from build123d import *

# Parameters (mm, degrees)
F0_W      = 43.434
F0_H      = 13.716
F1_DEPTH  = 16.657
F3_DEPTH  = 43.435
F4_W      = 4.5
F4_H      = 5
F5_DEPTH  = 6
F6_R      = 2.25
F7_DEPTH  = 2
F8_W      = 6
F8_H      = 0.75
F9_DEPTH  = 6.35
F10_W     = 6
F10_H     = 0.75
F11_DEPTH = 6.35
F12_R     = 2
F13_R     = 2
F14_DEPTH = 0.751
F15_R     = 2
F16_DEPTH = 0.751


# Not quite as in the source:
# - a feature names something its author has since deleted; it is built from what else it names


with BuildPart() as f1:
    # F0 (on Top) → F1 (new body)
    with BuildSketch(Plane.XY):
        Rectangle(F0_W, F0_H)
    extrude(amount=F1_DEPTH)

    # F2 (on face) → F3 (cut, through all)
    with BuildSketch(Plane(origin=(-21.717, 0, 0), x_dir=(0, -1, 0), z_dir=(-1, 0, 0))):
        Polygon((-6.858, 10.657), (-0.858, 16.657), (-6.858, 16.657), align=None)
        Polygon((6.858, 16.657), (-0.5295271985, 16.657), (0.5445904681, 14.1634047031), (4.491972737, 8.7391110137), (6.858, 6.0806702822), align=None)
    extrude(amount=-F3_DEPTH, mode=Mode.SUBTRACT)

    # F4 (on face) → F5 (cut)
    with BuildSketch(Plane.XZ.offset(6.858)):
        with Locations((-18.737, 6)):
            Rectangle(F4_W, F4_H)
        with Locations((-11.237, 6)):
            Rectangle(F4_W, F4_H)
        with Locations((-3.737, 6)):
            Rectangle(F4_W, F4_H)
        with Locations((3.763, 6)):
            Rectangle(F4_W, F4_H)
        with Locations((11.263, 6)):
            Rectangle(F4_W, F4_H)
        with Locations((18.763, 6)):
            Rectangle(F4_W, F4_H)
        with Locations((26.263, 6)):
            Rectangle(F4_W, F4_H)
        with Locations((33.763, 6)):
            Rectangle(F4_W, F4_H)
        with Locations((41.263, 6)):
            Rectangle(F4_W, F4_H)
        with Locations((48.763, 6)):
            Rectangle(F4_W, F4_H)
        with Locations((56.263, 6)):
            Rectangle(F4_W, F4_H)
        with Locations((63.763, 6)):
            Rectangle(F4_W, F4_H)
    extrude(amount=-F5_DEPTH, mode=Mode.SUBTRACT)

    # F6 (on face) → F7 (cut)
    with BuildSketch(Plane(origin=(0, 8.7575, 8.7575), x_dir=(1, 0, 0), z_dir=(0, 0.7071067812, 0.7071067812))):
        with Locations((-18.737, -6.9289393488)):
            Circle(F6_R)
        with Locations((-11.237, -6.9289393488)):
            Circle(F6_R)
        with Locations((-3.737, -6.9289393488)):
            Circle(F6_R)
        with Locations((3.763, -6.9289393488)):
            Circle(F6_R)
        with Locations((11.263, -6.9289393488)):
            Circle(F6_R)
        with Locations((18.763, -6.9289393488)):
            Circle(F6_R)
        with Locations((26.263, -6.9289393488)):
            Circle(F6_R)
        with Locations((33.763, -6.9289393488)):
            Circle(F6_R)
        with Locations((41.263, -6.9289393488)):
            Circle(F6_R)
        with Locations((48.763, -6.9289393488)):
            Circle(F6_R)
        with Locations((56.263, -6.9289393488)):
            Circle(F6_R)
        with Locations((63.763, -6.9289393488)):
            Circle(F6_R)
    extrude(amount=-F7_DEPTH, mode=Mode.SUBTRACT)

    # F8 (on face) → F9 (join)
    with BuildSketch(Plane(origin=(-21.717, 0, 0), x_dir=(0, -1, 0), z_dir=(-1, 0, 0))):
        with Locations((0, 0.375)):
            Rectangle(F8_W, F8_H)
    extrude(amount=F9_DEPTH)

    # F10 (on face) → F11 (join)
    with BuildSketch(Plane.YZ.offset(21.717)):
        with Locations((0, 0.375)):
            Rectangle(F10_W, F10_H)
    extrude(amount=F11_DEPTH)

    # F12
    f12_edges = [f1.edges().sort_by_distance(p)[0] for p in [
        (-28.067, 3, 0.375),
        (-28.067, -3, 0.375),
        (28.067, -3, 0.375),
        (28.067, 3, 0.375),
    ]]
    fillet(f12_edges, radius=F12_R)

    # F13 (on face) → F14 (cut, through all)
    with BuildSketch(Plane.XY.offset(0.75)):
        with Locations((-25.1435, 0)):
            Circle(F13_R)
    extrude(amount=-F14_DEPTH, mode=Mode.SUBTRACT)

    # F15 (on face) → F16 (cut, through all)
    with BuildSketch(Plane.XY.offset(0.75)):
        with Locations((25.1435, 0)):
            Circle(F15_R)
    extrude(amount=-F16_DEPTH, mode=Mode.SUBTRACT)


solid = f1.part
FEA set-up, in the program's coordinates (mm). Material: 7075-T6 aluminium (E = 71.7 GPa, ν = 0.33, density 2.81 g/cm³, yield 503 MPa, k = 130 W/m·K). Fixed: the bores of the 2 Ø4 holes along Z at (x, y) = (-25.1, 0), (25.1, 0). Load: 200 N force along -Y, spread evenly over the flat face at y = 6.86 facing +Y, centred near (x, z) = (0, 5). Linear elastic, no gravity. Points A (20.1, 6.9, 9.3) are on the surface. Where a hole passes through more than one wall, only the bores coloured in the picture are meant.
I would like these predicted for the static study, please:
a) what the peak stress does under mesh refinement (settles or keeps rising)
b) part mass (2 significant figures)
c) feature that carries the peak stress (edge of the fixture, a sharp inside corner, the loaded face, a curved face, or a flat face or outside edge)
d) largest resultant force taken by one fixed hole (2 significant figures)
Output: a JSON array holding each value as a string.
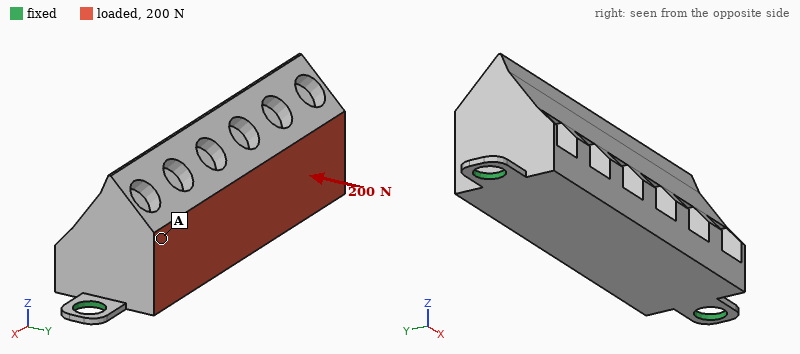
["keeps rising", "18 g", "edge of the fixture", "100 N"]
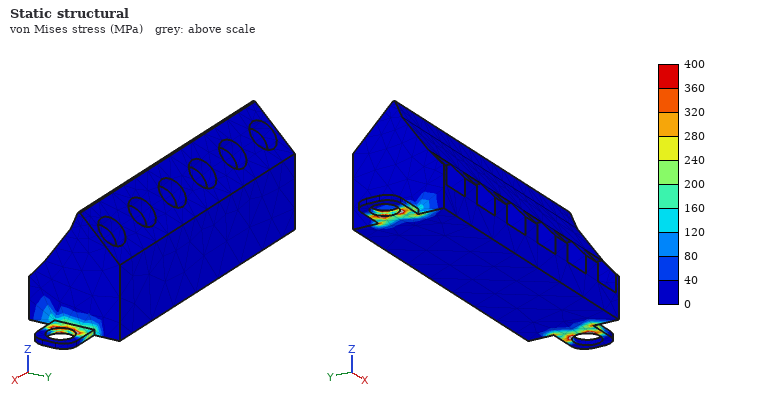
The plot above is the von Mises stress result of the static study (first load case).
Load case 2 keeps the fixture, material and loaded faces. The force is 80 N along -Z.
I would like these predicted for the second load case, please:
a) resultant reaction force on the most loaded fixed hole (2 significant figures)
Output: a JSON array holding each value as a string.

["50 N"]
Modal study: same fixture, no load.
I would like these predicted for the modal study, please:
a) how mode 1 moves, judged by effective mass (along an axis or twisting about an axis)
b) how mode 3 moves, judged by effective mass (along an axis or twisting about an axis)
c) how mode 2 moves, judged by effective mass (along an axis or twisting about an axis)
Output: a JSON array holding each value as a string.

["along Y", "along X", "along Z"]
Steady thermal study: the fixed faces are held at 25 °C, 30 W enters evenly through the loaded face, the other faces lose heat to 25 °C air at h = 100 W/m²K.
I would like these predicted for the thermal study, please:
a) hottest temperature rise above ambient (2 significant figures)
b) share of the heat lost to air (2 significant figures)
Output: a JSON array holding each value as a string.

["50 K", "43 %"]
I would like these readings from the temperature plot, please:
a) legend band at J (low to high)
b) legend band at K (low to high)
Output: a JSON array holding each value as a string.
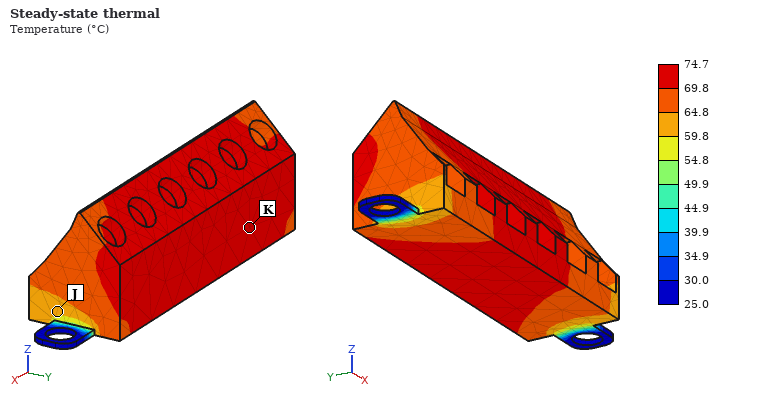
["59.8 to 64.8 °C", "69.8 to 74.7 °C"]
